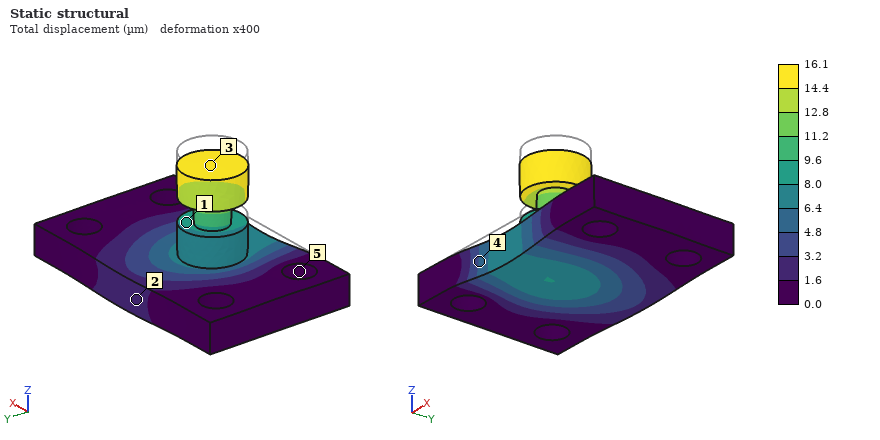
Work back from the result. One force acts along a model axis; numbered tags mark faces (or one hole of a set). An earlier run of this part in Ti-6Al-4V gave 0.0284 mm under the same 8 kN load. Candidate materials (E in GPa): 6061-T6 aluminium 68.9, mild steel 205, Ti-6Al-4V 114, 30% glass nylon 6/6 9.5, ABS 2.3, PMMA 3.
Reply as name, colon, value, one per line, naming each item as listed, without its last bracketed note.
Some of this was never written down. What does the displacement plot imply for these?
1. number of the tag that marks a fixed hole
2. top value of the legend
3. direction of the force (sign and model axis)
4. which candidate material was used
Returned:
number of the tag that marks a fixed hole: 5
top value of the legend: 16.1 µm
direction of the force: -Z
which candidate material was used: mild steel
